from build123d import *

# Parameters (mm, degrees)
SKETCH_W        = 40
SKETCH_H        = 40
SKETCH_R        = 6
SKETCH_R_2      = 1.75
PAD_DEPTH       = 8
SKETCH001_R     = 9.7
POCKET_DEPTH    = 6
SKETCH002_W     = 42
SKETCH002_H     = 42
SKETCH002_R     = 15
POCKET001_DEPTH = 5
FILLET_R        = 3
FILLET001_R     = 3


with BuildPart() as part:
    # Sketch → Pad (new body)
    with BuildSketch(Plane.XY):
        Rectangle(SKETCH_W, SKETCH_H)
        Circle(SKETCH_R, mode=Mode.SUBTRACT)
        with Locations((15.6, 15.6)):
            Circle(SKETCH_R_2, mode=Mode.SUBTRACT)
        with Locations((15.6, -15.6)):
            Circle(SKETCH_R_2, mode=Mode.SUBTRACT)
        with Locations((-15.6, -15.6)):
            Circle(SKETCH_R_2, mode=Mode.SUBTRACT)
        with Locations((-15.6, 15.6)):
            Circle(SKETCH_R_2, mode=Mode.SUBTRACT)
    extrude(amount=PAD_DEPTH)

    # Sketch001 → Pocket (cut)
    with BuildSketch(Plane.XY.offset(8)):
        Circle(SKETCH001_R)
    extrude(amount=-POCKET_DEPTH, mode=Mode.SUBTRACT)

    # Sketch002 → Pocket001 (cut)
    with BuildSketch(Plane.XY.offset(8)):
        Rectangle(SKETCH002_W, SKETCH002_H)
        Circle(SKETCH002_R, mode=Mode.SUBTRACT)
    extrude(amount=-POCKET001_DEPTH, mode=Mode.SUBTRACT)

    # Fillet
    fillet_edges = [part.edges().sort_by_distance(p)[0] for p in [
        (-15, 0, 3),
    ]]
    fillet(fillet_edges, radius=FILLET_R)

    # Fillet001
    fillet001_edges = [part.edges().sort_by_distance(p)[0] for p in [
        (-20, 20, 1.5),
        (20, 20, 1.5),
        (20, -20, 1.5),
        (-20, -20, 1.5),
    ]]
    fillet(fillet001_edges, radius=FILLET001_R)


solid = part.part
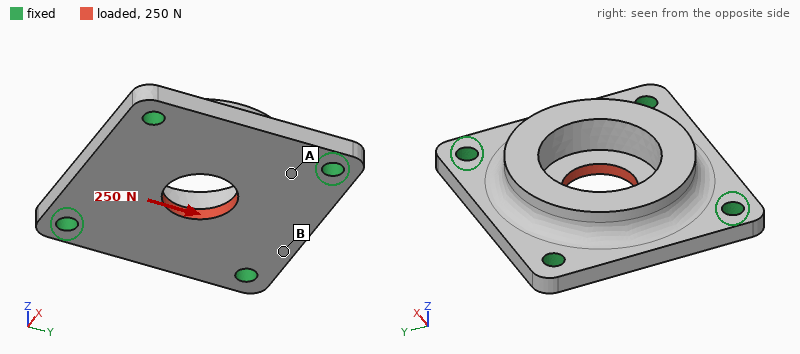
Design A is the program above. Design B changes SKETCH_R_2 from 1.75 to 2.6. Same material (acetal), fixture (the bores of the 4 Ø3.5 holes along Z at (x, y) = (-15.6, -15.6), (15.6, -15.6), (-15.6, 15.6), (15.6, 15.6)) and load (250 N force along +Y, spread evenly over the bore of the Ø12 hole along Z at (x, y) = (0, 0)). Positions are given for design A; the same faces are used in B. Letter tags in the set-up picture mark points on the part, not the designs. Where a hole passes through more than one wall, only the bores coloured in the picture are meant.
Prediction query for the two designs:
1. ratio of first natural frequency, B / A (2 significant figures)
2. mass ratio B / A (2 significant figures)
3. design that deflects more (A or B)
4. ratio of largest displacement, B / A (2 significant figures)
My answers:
1.2
0.98
A
0.92
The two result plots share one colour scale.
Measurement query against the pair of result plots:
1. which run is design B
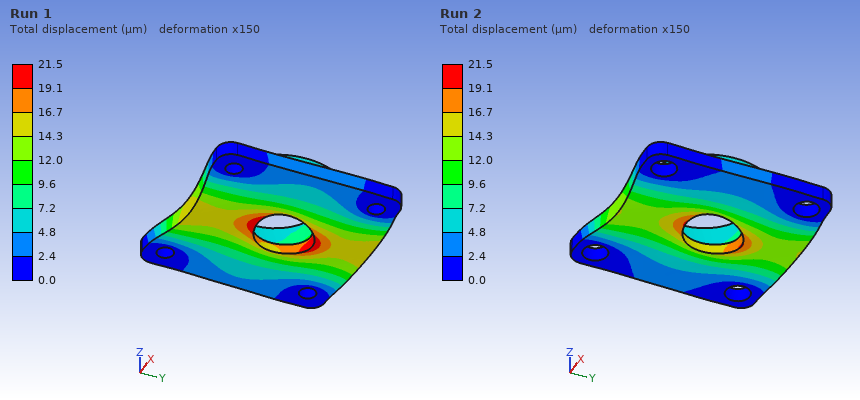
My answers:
Run 2
